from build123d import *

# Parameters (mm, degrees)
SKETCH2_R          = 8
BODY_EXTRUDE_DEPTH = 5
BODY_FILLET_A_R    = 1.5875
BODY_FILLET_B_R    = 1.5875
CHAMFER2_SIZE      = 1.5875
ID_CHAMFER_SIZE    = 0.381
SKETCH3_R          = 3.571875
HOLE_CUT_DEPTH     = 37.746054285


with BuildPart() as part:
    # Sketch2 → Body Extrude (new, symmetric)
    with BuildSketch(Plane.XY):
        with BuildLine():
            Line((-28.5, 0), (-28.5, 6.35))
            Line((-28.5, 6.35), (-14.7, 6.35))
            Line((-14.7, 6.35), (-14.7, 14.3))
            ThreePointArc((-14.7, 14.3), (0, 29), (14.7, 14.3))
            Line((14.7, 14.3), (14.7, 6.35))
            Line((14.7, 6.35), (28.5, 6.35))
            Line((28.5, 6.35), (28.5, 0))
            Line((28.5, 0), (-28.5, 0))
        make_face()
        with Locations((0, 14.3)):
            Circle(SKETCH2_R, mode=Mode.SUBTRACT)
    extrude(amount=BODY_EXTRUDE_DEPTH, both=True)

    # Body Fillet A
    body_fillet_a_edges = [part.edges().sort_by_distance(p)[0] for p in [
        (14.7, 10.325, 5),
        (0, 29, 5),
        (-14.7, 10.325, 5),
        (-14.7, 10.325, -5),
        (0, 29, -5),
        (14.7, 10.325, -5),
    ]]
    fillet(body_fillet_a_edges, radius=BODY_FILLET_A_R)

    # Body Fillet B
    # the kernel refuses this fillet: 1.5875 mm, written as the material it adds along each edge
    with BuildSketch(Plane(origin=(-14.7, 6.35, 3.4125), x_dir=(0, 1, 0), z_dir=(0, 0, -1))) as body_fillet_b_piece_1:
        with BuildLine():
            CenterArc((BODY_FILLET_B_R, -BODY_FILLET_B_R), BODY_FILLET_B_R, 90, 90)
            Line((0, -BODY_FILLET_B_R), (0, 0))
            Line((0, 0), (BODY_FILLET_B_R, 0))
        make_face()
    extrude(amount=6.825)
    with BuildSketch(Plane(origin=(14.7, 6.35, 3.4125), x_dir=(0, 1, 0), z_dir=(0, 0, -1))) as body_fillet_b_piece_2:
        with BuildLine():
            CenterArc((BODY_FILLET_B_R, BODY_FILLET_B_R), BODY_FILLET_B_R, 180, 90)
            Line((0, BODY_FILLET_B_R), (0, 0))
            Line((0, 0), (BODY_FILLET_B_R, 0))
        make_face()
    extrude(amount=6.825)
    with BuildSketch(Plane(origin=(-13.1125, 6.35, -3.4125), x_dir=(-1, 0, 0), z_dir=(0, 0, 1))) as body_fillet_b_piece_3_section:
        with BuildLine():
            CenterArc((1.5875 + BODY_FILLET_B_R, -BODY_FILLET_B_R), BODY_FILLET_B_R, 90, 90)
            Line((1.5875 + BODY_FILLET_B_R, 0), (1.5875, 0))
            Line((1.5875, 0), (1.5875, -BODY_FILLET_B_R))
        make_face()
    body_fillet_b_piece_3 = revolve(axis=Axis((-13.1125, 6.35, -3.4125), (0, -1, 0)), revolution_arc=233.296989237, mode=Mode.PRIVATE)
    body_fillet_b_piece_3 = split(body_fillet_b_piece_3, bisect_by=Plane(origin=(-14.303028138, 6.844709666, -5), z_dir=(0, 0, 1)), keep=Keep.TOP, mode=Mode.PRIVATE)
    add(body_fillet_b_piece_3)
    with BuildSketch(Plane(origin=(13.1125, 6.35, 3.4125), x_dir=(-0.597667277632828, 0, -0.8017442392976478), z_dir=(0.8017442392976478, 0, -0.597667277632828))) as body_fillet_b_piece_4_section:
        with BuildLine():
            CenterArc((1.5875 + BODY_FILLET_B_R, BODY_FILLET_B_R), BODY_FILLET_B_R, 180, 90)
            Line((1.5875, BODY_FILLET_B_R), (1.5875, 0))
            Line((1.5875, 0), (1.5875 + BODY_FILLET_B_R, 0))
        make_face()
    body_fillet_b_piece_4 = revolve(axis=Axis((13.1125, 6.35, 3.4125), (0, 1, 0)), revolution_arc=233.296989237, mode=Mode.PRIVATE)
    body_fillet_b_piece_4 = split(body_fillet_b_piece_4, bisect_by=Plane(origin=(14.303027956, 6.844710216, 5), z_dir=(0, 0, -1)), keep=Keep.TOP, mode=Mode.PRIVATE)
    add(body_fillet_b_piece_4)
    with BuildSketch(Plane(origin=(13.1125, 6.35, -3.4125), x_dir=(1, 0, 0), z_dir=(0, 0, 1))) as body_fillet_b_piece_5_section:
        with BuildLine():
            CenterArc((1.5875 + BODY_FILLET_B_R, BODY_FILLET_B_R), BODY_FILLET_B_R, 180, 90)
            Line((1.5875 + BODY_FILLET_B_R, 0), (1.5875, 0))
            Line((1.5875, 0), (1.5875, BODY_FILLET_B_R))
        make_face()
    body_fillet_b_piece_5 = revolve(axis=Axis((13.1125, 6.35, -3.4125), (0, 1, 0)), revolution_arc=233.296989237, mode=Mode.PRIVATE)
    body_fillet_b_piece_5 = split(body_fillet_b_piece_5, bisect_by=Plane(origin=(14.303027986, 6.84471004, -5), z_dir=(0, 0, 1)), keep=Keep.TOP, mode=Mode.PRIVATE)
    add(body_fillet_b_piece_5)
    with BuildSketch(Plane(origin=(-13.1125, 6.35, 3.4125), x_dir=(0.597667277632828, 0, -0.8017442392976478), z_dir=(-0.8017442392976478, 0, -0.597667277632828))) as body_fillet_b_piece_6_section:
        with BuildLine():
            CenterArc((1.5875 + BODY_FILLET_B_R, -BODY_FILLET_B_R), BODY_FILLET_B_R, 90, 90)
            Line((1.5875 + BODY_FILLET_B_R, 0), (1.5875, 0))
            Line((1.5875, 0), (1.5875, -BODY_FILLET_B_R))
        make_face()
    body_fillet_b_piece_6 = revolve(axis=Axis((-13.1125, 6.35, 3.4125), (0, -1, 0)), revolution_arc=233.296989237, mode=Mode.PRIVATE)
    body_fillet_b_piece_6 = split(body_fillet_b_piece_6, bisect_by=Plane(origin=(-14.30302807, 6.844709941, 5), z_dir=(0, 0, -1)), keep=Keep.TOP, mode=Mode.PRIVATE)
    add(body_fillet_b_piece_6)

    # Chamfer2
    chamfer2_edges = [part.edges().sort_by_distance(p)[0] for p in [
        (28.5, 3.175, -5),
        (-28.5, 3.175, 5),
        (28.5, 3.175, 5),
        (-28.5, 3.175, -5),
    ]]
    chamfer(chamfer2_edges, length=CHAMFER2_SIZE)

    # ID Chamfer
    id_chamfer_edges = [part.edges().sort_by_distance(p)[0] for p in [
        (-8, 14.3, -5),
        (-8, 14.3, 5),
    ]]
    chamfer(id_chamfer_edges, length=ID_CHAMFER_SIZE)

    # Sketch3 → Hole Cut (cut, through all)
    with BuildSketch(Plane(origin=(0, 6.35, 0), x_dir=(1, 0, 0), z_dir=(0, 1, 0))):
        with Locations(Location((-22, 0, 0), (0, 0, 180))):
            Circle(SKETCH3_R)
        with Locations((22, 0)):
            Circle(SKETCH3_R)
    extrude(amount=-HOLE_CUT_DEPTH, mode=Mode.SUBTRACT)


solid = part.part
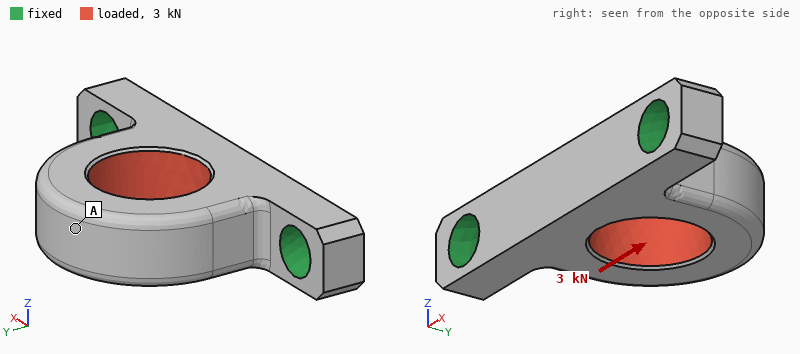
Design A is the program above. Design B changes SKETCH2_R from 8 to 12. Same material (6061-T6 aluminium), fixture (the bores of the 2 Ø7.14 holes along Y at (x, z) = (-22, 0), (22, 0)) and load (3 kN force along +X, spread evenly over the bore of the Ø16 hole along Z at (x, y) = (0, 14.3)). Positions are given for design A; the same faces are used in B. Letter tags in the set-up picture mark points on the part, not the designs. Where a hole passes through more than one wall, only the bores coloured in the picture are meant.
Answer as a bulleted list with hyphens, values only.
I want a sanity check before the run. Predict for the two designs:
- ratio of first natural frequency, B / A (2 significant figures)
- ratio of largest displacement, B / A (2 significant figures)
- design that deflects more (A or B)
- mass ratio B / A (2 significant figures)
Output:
- 1.2
- 9.1
- B
- 0.63
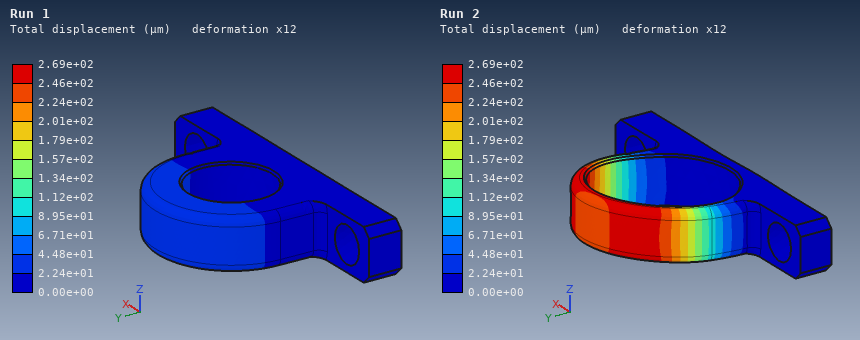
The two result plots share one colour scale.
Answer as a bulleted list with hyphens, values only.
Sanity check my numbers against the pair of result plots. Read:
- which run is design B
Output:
- Run 2
